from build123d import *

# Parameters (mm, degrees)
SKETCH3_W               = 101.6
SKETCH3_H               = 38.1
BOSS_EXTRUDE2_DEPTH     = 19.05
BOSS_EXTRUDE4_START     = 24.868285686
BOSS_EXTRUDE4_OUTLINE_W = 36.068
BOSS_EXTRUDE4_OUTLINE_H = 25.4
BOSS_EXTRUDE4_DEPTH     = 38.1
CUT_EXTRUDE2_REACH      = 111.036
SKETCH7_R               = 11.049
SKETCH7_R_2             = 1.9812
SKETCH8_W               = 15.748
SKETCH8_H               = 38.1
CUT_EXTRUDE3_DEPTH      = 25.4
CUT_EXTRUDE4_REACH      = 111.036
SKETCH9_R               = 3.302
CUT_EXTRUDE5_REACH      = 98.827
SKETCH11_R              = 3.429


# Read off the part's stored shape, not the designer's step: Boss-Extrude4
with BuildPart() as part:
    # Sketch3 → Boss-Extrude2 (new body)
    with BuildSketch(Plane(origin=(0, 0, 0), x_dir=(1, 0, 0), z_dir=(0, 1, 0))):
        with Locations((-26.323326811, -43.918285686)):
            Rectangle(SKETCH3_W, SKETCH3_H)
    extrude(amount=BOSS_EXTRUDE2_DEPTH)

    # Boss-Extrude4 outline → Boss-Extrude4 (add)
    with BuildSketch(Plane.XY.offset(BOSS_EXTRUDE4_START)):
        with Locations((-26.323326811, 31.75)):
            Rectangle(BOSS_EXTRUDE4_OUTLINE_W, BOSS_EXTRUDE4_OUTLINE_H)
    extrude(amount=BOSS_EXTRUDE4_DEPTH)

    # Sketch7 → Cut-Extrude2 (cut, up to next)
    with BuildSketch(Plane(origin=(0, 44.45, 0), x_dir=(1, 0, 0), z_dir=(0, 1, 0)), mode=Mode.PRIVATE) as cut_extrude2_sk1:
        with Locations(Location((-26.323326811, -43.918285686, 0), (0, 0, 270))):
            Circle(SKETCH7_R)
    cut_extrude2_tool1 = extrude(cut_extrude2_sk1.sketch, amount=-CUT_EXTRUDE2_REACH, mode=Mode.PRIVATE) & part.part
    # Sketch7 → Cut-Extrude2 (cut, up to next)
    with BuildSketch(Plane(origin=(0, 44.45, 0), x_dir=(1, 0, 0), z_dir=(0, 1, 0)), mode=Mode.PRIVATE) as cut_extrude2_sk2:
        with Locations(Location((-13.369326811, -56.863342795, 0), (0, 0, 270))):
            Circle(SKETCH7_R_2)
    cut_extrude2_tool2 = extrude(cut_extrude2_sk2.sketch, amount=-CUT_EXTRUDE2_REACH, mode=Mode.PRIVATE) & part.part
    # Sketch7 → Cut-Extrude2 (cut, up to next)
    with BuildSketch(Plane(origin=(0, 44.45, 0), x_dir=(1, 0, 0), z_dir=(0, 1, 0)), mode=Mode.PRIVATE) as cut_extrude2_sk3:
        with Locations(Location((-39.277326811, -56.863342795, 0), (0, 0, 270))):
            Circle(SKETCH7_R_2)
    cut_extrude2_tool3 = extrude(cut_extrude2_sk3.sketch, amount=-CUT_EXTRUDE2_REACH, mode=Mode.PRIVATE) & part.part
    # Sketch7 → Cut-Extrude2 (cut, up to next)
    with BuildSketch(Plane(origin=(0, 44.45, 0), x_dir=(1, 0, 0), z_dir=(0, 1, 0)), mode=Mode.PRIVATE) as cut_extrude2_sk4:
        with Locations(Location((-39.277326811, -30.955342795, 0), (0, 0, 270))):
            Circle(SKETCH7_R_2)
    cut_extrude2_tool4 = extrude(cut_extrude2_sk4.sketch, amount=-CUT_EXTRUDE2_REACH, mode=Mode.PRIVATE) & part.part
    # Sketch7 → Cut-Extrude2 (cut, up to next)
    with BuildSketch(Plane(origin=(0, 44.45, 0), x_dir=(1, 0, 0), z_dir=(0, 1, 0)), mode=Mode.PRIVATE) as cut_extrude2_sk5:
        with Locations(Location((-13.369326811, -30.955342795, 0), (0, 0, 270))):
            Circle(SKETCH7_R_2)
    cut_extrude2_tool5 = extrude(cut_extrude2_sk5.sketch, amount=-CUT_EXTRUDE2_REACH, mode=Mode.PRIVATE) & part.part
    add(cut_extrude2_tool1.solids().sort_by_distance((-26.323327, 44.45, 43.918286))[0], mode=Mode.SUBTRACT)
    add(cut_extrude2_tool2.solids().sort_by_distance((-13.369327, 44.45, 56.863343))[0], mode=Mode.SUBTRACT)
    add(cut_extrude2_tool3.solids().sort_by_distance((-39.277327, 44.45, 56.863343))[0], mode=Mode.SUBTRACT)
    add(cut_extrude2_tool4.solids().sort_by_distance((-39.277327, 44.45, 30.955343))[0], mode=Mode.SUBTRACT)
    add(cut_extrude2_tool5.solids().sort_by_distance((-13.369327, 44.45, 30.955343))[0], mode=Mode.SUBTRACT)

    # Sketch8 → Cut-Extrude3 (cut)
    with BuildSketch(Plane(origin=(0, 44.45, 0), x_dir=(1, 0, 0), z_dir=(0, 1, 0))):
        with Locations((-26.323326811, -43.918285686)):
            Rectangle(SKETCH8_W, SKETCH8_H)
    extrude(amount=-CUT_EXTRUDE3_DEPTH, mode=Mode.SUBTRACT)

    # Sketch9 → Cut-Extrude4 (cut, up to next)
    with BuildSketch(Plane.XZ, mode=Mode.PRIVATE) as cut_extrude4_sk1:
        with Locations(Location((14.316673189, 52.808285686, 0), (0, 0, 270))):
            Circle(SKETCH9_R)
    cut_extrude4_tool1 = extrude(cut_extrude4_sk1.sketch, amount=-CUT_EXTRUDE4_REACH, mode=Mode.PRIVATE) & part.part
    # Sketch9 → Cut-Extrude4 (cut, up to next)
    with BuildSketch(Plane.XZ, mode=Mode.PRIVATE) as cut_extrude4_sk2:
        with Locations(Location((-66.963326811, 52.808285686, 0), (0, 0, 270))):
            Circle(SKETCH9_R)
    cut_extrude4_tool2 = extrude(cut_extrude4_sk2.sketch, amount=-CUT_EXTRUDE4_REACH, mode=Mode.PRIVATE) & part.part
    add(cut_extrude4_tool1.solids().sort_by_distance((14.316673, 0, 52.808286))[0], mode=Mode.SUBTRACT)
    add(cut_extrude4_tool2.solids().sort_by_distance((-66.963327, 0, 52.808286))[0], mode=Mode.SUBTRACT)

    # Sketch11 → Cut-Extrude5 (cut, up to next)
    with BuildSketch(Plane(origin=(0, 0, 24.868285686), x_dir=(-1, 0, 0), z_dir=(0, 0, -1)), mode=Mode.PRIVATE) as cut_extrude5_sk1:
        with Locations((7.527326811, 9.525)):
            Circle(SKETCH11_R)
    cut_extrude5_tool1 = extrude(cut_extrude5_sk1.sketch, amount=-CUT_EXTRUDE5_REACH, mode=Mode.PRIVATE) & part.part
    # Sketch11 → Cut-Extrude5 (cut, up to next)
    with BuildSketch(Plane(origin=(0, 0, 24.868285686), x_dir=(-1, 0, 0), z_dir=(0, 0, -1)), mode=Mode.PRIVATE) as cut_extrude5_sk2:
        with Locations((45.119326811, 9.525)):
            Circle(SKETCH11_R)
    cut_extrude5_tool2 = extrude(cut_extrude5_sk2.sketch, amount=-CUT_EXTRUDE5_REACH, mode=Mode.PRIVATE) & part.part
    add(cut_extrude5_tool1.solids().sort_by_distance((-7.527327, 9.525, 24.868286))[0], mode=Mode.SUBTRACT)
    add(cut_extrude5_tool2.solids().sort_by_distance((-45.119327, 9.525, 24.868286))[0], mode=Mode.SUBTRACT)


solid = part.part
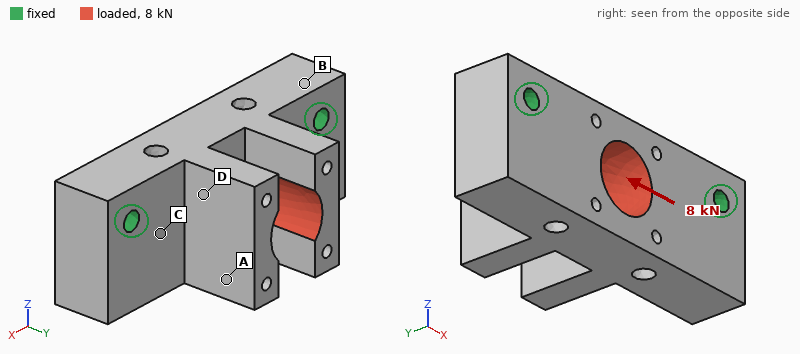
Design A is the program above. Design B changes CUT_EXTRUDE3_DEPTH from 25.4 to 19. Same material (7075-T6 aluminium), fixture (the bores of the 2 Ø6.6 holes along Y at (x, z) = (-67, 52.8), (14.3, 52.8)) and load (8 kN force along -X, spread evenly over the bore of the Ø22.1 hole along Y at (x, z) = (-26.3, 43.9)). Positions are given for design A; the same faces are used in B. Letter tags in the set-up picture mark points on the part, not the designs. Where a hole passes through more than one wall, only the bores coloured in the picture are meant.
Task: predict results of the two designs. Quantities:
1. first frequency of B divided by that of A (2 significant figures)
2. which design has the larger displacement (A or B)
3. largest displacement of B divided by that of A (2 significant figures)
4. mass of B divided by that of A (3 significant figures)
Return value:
1.0
A
0.70
1.02
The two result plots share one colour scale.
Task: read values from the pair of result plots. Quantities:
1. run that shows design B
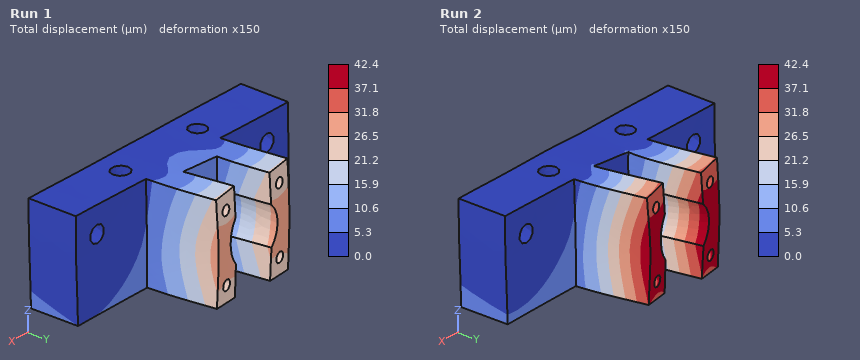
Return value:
Run 1
